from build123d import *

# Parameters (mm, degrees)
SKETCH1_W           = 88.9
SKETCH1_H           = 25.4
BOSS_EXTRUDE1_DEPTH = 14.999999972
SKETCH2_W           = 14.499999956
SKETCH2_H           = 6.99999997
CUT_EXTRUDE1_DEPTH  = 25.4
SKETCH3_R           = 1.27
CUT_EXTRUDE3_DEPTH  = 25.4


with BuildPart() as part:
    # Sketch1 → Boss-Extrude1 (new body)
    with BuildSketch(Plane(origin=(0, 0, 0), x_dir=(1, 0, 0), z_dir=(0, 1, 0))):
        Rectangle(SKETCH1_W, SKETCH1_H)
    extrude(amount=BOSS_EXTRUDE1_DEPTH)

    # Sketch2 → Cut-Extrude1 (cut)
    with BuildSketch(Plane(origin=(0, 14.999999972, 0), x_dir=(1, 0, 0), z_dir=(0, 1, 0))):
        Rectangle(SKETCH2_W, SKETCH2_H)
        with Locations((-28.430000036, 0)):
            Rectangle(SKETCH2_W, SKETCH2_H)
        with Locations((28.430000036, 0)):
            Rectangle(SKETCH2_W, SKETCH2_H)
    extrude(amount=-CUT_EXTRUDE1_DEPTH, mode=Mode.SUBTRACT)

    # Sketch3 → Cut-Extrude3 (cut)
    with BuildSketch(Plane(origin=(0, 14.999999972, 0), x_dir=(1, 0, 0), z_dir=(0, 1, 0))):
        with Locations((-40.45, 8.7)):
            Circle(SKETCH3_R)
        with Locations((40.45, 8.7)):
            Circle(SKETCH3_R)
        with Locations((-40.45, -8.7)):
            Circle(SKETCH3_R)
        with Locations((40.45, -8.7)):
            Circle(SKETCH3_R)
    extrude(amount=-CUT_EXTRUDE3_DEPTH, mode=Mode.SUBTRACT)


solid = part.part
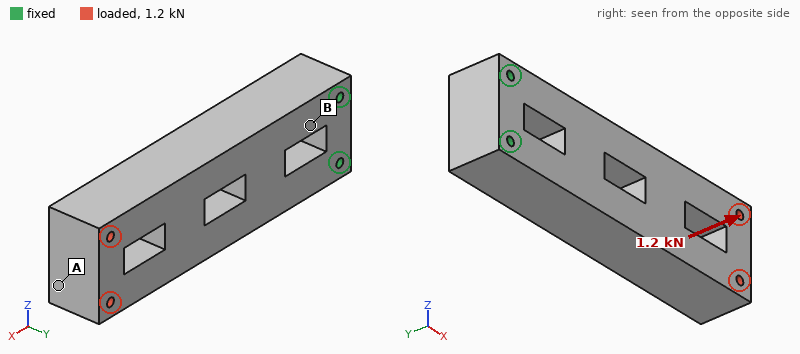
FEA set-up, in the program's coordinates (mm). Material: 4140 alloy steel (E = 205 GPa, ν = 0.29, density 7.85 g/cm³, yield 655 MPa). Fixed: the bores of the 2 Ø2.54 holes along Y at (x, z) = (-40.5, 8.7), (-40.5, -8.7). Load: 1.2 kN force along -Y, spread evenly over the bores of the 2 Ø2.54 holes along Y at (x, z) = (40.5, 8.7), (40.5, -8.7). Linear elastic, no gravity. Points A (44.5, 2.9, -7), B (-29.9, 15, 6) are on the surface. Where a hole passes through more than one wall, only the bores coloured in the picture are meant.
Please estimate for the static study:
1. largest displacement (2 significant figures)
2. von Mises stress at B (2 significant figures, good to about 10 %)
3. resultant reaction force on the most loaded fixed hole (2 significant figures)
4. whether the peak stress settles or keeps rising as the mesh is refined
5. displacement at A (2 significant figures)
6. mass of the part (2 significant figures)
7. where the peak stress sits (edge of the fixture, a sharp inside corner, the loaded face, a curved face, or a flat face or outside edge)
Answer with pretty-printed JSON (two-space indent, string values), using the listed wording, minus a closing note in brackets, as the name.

{
  "largest displacement": "0.22 mm",
  "von Mises stress at B": "120 MPa",
  "resultant reaction force on the most loaded fixed hole": "600 N",
  "whether the peak stress settles or keeps rising as the mesh is refined": "keeps rising",
  "displacement at A": "0.21 mm",
  "mass of the part": "230 g",
  "where the peak stress sits": "edge of the fixture"
}
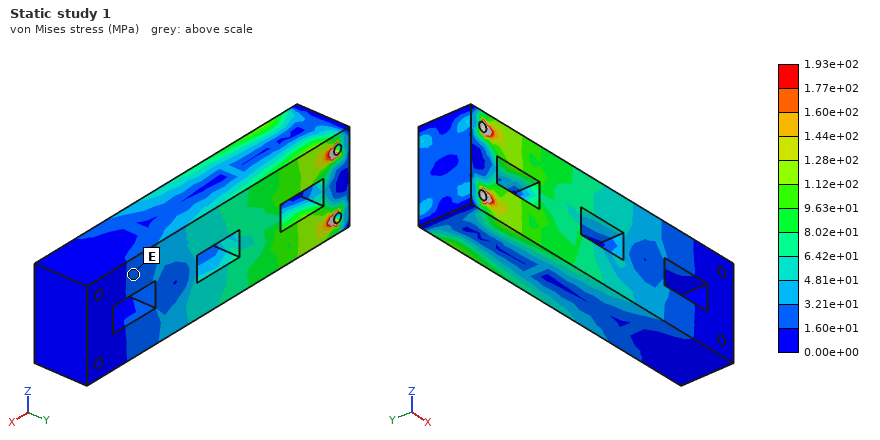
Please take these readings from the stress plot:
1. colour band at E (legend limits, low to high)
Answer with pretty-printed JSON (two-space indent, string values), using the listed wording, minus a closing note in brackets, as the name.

{
  "colour band at E": "1.60e+01 to 3.21e+01 MPa"
}
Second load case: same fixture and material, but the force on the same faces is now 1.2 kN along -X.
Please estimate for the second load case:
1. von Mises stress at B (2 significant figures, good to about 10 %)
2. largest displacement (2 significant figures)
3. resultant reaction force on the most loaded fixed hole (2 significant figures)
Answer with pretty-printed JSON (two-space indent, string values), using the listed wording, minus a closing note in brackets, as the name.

{
  "von Mises stress at B": "4.3 MPa",
  "largest displacement": "1.8 µm",
  "resultant reaction force on the most loaded fixed hole": "600 N"
}
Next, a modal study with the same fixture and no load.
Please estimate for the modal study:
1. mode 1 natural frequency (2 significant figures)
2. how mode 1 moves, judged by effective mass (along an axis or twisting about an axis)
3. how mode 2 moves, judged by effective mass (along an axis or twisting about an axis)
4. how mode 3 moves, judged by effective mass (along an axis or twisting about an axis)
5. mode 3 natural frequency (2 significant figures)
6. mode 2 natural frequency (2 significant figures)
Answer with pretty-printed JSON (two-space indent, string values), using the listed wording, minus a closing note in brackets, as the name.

{
  "mode 1 natural frequency": "1600 Hz",
  "how mode 1 moves, judged by effective mass": "along Y",
  "how mode 2 moves, judged by effective mass": "along Z",
  "how mode 3 moves, judged by effective mass": "twisting about X",
  "mode 3 natural frequency": "6400 Hz",
  "mode 2 natural frequency": "2600 Hz"
}
